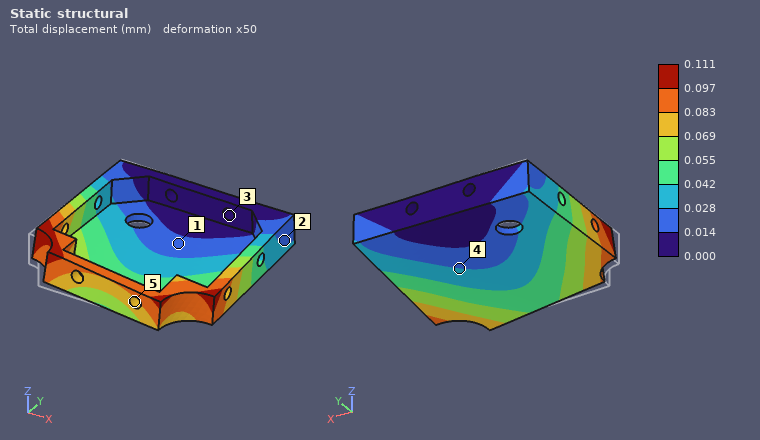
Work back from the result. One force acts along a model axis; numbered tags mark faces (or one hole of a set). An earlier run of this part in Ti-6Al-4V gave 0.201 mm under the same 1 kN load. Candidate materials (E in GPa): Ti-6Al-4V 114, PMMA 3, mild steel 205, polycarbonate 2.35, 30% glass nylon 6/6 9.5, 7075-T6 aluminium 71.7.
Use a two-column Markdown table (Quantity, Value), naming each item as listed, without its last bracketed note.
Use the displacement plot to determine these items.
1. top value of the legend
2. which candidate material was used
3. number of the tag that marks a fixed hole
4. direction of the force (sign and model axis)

| Quantity | Value |
|---|---|
| top value of the legend | 0.111 mm |
| which candidate material was used | mild steel |
| number of the tag that marks a fixed hole | 3 |
| direction of the force | +X |
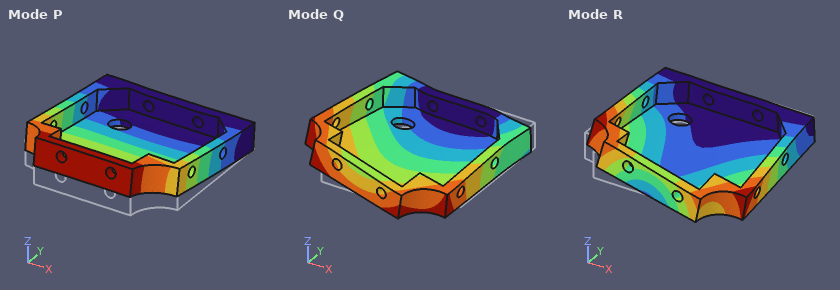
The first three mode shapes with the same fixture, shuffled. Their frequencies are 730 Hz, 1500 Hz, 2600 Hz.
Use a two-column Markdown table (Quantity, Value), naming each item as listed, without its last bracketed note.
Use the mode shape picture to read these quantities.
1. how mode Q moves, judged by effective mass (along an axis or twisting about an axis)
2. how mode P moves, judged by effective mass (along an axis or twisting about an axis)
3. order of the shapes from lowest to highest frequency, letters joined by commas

| Quantity | Value |
|---|---|
| how mode Q moves, judged by effective mass | along X |
| how mode P moves, judged by effective mass | along Z |
| order of the shapes from lowest to highest frequency, letters joined by commas | P, R, Q |
